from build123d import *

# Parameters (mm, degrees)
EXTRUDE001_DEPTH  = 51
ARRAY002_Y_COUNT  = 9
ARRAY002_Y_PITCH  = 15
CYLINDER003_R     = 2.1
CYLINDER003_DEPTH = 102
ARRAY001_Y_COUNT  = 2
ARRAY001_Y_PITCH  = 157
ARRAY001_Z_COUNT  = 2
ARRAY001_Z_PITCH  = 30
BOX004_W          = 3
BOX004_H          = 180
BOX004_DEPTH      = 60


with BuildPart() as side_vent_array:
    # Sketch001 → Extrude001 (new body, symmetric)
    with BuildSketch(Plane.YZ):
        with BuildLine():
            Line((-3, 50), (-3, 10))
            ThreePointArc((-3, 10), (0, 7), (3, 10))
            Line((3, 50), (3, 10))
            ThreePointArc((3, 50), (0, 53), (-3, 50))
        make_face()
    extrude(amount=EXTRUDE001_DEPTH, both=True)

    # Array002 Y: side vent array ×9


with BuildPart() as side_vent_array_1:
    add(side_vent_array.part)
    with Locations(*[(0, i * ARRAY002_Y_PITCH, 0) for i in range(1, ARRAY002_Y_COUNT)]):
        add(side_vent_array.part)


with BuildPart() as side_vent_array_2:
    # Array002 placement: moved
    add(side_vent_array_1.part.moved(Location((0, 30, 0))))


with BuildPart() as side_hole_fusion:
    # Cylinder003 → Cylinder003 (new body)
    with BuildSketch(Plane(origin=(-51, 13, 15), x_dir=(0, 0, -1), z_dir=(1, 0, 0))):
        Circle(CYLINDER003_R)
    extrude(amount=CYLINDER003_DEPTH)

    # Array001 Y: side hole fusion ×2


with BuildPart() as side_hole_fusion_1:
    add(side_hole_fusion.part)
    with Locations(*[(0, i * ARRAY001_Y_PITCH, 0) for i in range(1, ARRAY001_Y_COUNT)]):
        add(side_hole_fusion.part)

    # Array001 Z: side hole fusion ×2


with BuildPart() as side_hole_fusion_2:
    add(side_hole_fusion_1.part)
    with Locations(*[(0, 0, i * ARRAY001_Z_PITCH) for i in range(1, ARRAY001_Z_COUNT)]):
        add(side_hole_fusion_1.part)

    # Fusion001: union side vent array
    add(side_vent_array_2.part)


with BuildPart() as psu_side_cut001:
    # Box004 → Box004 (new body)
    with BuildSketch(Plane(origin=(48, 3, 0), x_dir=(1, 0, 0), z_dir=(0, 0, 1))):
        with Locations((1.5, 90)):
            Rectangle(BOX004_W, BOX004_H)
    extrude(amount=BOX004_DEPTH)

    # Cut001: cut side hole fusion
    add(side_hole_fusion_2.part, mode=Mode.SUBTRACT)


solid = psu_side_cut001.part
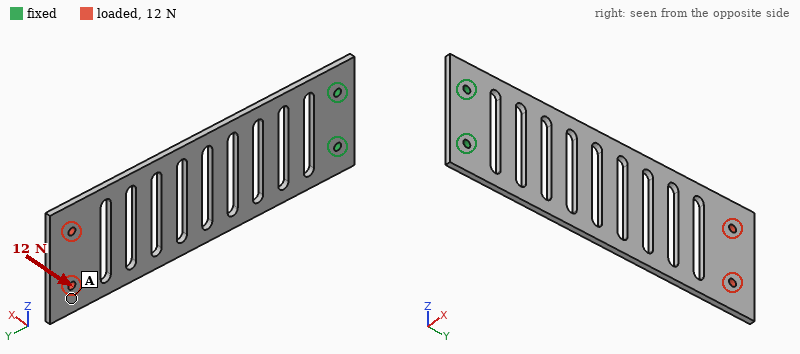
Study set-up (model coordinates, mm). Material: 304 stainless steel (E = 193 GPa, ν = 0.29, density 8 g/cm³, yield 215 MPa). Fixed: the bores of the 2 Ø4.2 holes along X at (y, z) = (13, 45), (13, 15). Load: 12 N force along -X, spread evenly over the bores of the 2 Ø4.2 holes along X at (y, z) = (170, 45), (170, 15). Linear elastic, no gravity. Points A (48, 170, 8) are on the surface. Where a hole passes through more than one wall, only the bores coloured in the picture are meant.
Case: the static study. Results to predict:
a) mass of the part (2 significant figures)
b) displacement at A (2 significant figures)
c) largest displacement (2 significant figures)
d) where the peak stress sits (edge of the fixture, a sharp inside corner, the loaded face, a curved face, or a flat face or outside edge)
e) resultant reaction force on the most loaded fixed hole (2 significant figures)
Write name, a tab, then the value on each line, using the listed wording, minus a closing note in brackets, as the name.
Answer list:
mass of the part	200 g
displacement at A	1.9 mm
largest displacement	2.2 mm
where the peak stress sits	a curved face
resultant reaction force on the most loaded fixed hole	6.0 N
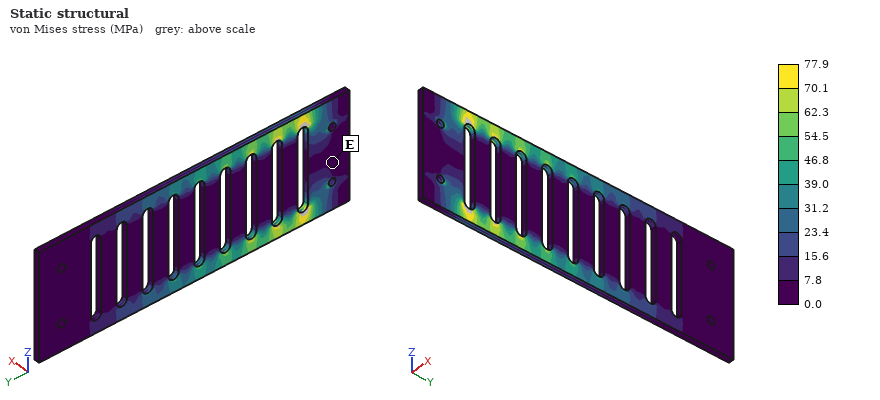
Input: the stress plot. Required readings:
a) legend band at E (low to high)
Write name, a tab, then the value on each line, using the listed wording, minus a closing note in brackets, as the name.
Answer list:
legend band at E	0.0 to 7.8 MPa
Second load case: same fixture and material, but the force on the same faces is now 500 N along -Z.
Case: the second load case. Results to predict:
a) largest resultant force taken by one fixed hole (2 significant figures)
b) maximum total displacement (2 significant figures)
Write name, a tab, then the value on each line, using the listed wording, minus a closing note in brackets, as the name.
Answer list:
largest resultant force taken by one fixed hole	2.3 kN
maximum total displacement	0.27 mm
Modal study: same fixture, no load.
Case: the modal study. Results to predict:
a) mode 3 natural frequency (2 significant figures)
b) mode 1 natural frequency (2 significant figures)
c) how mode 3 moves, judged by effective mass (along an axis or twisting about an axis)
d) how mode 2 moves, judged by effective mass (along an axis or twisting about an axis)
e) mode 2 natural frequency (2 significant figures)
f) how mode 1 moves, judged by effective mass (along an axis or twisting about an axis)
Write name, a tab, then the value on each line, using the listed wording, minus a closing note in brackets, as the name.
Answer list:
mode 3 natural frequency	400 Hz
mode 1 natural frequency	51 Hz
how mode 3 moves, judged by effective mass	twisting about Y
how mode 2 moves, judged by effective mass	along X
mode 2 natural frequency	330 Hz
how mode 1 moves, judged by effective mass	along X
